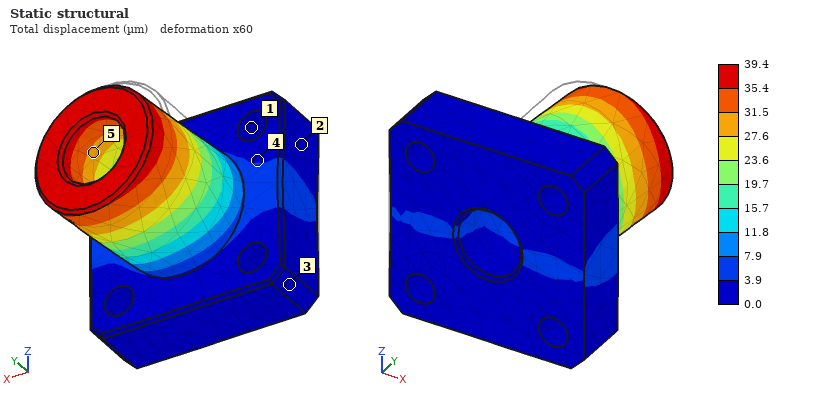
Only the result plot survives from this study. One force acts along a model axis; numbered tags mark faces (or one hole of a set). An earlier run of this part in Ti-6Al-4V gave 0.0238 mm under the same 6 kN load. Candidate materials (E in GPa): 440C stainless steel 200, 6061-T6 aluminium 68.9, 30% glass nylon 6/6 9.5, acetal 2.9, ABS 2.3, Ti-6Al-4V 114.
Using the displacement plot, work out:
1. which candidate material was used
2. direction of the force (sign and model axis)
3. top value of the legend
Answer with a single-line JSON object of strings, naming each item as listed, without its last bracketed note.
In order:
{"which candidate material was used": "6061-T6 aluminium", "direction of the force": "+X", "top value of the legend": "39.4 µm"}
